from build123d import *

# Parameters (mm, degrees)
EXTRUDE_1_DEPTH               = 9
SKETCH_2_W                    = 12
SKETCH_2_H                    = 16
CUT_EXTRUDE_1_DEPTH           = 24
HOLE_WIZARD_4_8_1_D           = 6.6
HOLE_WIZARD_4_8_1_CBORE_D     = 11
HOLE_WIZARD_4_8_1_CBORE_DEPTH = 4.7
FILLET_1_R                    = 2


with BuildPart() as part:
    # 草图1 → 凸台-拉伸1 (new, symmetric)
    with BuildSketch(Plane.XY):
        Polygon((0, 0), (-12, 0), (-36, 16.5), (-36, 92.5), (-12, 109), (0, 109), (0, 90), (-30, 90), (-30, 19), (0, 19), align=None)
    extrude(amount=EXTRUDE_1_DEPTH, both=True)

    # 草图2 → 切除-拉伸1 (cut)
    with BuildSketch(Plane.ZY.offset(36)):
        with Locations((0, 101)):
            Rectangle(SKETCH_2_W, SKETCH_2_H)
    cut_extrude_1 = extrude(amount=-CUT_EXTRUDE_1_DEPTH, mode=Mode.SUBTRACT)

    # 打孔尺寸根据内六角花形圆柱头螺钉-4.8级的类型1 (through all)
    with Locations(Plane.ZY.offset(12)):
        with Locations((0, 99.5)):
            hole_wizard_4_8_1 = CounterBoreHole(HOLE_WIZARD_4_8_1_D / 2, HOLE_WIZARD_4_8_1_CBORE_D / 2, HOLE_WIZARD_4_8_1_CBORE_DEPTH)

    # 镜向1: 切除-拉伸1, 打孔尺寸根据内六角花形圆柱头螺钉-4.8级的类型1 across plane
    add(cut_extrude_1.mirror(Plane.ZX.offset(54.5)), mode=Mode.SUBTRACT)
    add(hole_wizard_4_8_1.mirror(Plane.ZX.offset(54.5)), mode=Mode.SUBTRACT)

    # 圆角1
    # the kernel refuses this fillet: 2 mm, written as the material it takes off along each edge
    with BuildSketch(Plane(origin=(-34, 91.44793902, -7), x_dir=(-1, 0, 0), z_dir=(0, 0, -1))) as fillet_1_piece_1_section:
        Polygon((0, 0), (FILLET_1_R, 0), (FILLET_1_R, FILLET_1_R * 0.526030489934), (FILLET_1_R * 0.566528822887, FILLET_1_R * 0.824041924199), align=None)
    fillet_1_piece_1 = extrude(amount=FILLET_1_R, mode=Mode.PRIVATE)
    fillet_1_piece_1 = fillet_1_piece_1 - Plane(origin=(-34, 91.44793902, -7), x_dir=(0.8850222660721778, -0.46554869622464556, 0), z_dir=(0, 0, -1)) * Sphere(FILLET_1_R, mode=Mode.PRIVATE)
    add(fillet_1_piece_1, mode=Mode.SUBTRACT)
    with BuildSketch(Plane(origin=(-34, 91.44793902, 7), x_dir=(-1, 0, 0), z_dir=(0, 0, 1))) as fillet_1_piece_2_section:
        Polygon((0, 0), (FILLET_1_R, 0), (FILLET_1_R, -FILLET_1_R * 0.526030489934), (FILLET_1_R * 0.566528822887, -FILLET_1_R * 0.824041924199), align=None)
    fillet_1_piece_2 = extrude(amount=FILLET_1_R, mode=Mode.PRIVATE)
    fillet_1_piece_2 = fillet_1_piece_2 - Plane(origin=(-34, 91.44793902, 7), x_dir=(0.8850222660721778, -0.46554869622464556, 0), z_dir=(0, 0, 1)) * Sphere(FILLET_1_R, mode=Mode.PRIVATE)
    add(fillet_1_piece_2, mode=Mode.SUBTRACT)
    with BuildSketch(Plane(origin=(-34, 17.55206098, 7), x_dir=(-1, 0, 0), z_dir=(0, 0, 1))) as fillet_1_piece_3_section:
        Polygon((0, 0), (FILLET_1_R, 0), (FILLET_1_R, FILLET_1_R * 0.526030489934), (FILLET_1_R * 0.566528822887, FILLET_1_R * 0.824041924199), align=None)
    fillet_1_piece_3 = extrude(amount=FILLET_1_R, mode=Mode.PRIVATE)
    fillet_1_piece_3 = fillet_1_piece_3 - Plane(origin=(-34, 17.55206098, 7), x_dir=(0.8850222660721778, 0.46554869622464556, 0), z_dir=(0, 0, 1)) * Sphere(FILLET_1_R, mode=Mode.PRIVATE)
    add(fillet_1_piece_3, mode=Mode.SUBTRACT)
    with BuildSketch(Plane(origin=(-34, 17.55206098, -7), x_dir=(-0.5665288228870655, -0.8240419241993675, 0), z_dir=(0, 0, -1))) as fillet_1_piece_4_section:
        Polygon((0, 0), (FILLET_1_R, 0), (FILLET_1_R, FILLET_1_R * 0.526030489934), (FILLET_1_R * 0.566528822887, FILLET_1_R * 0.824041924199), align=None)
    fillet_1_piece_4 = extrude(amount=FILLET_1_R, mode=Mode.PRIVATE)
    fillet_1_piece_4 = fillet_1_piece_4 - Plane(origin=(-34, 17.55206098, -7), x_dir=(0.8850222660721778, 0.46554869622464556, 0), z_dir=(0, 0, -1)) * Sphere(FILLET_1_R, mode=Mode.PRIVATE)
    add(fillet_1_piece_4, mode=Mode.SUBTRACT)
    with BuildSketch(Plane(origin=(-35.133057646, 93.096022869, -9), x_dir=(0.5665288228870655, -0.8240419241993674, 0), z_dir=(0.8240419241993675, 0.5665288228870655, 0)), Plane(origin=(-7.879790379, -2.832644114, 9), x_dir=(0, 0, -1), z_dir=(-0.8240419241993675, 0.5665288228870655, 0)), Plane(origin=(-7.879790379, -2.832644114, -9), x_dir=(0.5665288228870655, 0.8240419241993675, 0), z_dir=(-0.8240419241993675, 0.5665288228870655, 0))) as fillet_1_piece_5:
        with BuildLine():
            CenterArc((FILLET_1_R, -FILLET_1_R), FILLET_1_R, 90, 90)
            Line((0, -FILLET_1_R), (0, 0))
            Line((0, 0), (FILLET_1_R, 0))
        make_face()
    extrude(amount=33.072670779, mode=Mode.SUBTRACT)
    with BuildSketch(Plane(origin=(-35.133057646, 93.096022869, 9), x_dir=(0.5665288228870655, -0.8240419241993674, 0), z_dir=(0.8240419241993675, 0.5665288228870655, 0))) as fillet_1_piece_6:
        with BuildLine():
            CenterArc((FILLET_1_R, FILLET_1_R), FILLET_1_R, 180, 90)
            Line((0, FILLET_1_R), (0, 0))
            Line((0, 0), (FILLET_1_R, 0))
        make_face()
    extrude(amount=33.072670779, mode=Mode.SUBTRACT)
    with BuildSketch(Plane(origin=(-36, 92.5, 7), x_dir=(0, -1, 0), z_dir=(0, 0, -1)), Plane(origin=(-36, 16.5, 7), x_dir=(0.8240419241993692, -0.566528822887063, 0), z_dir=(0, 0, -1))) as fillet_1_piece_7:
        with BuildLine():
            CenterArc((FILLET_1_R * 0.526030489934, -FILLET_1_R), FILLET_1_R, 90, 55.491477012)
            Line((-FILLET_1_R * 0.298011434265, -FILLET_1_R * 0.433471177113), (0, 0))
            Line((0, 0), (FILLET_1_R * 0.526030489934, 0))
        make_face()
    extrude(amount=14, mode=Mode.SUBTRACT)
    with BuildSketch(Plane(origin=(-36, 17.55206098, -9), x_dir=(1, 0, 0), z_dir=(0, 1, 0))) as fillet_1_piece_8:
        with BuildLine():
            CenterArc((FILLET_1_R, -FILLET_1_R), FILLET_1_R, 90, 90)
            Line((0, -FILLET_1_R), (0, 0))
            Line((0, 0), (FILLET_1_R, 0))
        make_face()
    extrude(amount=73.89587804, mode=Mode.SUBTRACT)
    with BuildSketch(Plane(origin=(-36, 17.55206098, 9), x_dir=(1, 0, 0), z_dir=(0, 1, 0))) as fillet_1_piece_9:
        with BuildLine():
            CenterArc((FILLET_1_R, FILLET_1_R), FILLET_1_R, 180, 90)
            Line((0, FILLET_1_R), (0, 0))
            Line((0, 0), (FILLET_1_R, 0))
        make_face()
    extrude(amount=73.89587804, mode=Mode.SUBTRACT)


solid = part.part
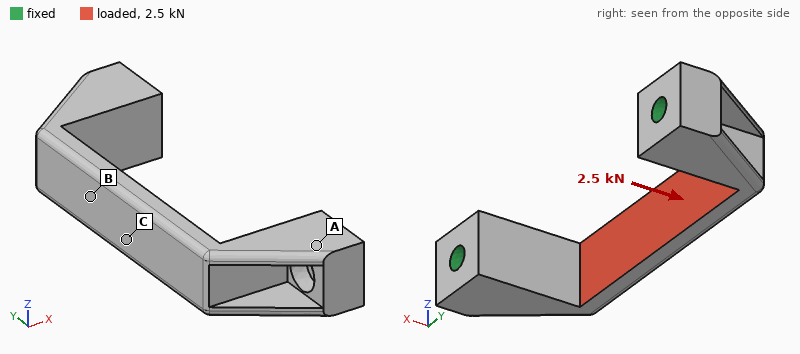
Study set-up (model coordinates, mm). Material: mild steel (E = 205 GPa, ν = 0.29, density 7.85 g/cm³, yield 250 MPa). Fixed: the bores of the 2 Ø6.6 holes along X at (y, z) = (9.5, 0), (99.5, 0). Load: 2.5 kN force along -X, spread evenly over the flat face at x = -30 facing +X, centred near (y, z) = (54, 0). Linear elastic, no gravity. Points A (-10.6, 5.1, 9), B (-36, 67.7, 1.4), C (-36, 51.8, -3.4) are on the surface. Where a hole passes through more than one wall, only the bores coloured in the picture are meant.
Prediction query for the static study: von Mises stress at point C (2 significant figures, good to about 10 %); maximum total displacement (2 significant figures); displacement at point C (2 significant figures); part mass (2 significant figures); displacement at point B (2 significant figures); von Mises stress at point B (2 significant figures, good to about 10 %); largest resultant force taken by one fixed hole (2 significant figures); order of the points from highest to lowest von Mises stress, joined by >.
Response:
120 MPa
87 µm
84 µm
150 g
70 µm
91 MPa
1.6 kN
C > B > A
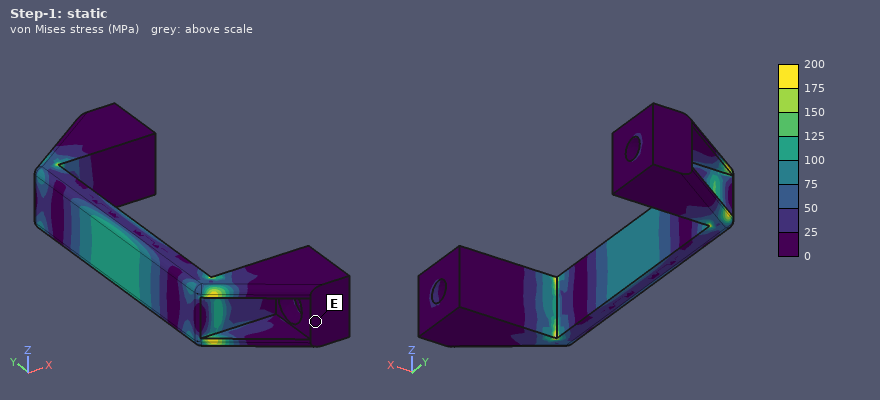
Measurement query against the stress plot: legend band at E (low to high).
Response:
0 to 25 MPa
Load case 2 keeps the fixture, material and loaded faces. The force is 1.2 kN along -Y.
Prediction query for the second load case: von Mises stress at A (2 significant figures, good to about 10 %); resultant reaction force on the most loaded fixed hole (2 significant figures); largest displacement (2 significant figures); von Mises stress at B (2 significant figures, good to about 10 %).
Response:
18 MPa
600 N
15 µm
6.7 MPa
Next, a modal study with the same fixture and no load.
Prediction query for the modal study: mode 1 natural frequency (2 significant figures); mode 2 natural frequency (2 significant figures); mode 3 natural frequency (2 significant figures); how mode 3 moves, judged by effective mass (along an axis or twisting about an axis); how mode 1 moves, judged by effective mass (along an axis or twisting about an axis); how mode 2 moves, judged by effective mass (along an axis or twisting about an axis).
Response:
4000 Hz
4500 Hz
5400 Hz
along Y
along X
along Z
